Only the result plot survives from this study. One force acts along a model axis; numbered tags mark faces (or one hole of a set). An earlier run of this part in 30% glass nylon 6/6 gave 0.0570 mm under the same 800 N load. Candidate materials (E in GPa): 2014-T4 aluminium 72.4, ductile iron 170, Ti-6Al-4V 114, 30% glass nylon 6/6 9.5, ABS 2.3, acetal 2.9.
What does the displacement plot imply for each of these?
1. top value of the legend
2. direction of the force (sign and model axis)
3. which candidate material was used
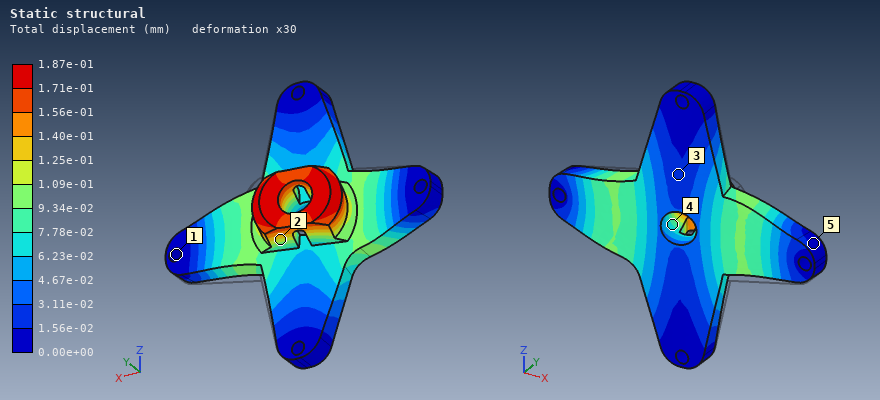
1.87e-01 mm
-X
acetal
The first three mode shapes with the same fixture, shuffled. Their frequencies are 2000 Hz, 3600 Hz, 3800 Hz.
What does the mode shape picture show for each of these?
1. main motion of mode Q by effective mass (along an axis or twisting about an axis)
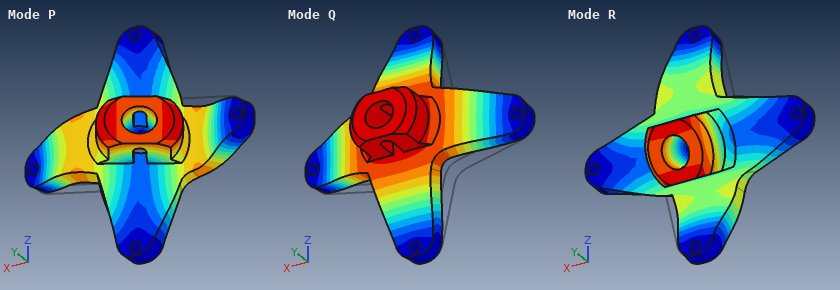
along Y
